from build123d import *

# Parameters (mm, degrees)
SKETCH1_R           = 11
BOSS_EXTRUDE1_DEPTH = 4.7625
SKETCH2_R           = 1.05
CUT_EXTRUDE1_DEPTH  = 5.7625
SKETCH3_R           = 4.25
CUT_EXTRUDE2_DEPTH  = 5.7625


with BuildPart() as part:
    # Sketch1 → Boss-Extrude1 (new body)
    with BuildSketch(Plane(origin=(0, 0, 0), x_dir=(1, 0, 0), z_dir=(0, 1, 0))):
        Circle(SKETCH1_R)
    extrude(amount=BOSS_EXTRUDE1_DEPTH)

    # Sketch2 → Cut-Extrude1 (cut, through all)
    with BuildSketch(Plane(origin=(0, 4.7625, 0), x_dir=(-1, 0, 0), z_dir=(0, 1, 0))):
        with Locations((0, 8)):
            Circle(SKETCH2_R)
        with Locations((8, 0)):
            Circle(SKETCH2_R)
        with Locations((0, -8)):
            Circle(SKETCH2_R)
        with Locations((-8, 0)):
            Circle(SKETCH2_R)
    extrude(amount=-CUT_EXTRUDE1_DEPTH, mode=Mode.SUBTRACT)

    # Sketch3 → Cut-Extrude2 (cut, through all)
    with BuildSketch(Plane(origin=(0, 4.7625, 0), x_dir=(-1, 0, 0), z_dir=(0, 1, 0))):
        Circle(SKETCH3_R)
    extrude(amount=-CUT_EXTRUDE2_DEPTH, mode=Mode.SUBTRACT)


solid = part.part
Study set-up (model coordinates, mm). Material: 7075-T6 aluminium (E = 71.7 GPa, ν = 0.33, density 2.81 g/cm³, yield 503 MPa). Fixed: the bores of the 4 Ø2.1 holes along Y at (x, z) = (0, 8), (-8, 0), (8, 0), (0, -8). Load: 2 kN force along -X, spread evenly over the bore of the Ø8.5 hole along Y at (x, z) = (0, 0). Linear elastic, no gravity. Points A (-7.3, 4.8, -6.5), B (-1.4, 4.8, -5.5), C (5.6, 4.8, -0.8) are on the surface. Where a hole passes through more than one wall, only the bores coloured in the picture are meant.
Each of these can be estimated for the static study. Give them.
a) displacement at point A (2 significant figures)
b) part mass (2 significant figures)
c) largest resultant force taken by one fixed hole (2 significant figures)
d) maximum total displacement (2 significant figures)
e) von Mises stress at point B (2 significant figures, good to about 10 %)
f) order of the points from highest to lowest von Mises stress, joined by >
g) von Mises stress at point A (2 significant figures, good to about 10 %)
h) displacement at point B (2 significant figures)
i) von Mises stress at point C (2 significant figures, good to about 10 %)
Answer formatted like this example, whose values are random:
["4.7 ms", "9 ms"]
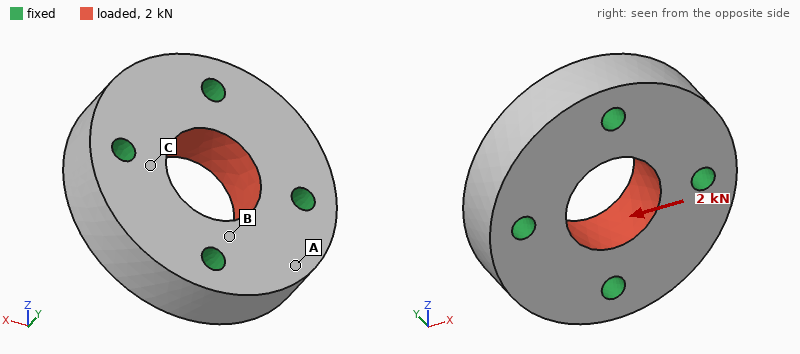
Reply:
["0.95 µm", "4.1 g", "560 N", "1.7 µm", "12 MPa", "C > B > A", "6.7 MPa", "1.0 µm", "24 MPa"]
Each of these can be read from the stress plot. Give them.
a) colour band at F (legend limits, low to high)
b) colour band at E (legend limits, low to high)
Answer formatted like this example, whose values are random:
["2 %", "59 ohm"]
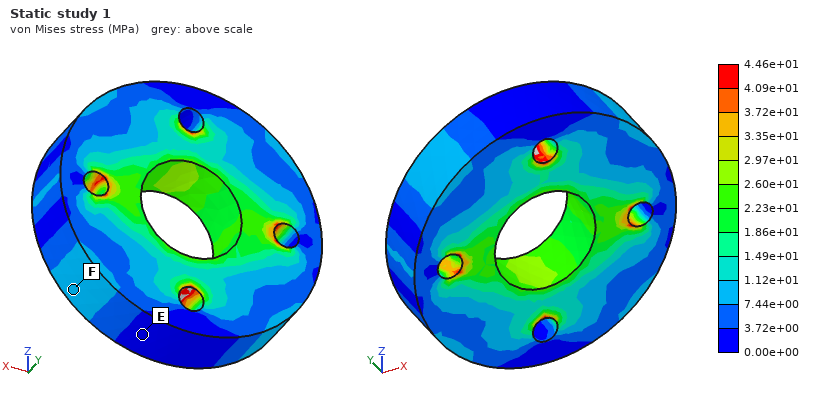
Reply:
["7.44e+00 to 1.12e+01 MPa", "0.00e+00 to 3.72e+00 MPa"]
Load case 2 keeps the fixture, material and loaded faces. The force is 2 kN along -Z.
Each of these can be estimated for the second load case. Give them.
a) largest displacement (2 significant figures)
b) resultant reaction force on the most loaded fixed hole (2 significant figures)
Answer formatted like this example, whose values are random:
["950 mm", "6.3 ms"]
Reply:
["1.7 µm", "560 N"]
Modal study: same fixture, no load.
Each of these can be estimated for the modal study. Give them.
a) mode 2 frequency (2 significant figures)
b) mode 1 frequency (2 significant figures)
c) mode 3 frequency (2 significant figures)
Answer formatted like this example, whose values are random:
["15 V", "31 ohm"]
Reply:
["85 kHz", "81 kHz", "85 kHz"]
